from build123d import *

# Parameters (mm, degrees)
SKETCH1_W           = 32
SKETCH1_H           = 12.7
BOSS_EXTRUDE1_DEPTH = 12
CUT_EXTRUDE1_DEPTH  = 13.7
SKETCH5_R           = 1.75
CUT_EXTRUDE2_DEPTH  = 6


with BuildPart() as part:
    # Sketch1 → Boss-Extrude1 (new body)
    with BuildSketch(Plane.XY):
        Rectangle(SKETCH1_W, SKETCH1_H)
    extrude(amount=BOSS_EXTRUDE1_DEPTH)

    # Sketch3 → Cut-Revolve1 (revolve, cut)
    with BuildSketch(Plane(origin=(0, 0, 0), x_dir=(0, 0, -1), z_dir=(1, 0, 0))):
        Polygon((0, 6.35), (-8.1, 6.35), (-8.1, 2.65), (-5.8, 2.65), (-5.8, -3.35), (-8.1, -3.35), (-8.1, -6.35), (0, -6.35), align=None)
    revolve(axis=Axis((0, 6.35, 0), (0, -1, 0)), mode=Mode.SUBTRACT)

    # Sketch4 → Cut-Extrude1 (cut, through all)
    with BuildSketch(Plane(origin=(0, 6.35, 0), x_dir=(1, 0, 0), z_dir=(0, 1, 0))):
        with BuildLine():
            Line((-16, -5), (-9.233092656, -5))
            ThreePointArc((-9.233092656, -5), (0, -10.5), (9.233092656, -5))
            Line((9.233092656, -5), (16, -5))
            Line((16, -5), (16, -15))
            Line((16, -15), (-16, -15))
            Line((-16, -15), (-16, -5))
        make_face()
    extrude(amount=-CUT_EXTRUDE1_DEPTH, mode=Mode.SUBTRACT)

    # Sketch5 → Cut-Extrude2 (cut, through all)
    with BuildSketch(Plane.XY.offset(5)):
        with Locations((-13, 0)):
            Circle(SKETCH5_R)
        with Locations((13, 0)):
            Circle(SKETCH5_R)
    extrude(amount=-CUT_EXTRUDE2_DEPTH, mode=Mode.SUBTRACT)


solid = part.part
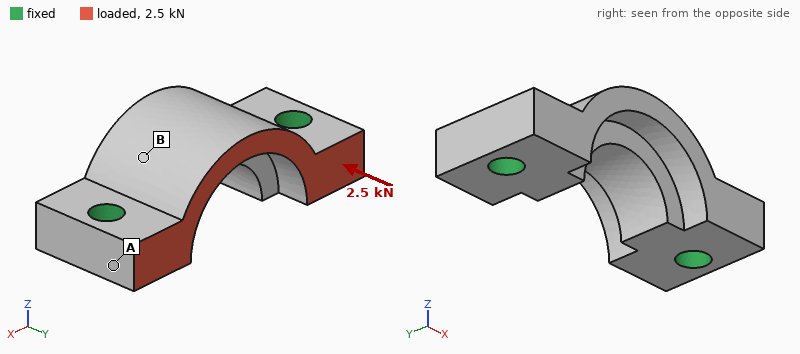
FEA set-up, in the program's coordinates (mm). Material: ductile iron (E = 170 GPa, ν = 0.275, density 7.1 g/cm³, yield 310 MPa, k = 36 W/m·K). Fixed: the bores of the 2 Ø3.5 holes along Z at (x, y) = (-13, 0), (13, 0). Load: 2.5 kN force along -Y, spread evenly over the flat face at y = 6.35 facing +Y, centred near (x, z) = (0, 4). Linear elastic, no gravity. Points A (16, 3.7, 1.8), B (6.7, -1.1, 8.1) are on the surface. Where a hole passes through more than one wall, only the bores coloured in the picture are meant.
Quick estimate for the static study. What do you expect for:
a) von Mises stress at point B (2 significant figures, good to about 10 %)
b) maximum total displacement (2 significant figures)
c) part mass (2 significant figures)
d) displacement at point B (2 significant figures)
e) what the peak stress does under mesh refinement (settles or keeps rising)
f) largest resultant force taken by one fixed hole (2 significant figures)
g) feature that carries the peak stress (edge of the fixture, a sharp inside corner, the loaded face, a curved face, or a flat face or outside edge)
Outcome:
39 MPa
11 µm
13 g
5.5 µm
keeps rising
1.3 kN
edge of the fixture
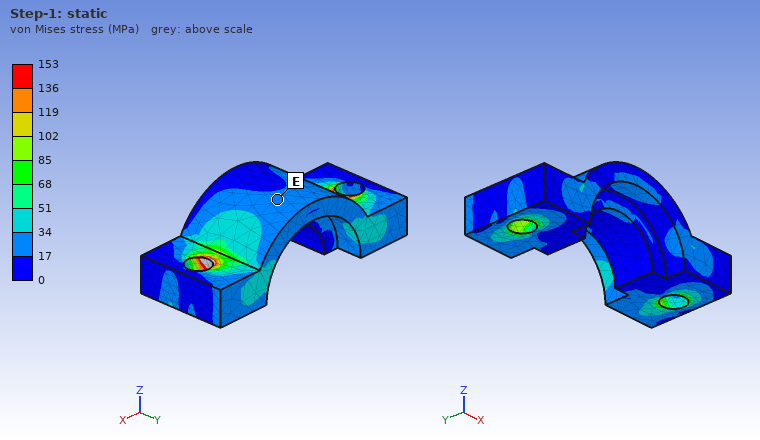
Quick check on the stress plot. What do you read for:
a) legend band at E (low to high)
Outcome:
17 to 34 MPa
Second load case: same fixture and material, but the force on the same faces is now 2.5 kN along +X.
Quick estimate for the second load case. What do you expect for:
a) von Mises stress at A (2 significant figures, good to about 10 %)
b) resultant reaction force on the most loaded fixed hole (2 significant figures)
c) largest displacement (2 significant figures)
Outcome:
43 MPa
1.3 kN
6.6 µm
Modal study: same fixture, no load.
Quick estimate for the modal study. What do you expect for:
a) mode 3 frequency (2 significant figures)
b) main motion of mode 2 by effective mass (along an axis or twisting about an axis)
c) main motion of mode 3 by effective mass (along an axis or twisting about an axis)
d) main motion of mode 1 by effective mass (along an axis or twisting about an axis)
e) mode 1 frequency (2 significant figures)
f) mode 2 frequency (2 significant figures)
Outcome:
54 kHz
along Z
along X
along Y
25 kHz
43 kHz
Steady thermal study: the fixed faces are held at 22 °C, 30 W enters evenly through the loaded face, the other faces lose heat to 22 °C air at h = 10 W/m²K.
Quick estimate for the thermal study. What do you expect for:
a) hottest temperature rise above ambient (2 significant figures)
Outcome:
68 K
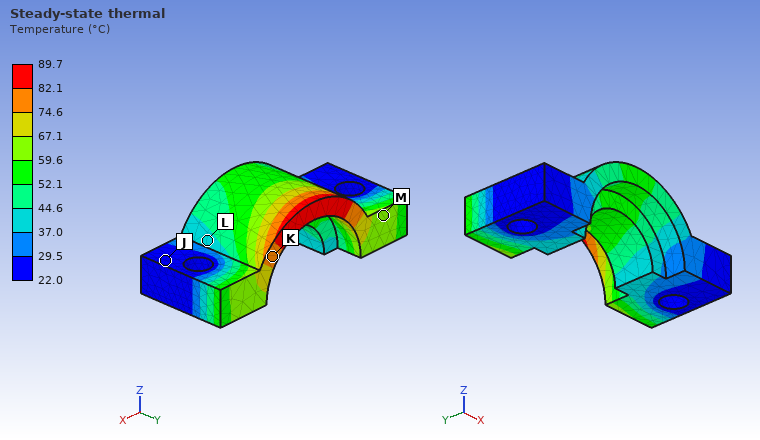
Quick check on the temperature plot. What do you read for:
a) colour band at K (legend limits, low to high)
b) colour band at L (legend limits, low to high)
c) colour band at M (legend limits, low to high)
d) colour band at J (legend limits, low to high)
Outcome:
74.6 to 82.1 °C
37.0 to 44.6 °C
59.6 to 67.1 °C
22.0 to 29.5 °C
